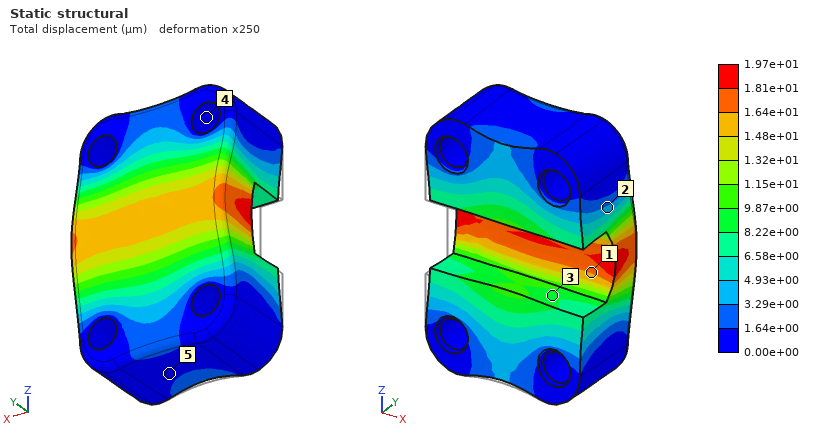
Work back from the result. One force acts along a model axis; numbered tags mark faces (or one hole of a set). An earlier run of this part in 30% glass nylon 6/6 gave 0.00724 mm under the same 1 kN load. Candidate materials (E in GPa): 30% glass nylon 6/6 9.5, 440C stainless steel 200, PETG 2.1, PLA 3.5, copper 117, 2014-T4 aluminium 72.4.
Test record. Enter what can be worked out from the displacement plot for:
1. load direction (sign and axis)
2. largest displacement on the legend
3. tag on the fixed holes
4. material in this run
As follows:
+Y
1.97e+01 µm
4
PLA
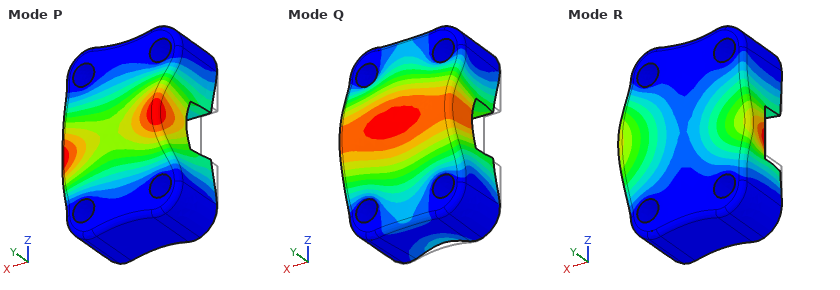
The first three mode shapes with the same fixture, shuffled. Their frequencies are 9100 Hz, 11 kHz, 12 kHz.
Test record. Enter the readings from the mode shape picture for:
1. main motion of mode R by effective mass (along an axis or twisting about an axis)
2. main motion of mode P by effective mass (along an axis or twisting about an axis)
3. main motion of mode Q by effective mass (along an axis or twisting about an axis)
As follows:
along X
along X
along Y
